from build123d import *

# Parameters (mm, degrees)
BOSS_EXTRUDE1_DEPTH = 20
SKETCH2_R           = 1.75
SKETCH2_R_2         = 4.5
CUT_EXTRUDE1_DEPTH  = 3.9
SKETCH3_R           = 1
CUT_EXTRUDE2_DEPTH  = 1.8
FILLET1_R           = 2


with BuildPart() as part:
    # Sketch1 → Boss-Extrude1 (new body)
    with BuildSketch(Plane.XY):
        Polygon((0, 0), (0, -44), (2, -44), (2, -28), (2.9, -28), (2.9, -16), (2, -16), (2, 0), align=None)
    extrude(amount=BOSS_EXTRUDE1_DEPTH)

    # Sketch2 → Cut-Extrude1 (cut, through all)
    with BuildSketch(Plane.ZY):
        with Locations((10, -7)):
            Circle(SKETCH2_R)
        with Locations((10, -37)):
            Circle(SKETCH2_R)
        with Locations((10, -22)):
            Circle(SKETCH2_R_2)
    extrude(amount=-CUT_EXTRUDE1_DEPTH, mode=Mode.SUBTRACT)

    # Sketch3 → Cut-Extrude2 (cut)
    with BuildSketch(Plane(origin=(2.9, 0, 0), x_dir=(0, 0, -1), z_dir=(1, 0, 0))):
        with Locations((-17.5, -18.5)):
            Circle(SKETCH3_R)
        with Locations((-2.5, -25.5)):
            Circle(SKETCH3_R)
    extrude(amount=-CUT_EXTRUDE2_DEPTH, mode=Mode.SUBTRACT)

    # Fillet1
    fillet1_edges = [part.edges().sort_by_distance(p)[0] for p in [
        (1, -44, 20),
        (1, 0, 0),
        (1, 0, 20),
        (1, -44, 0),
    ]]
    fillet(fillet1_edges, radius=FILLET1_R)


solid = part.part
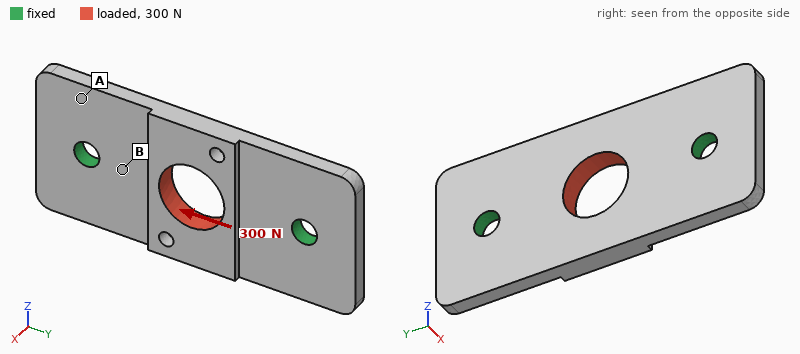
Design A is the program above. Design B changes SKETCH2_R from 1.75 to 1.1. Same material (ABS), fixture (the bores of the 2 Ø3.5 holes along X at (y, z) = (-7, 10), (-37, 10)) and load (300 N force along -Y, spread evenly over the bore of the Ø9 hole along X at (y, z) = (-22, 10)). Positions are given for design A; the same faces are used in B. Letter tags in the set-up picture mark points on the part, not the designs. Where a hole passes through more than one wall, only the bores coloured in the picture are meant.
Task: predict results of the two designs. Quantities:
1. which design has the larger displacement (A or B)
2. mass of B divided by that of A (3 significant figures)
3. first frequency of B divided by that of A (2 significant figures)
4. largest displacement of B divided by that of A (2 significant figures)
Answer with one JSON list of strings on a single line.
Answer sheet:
["B", "1.01", "0.86", "1.1"]
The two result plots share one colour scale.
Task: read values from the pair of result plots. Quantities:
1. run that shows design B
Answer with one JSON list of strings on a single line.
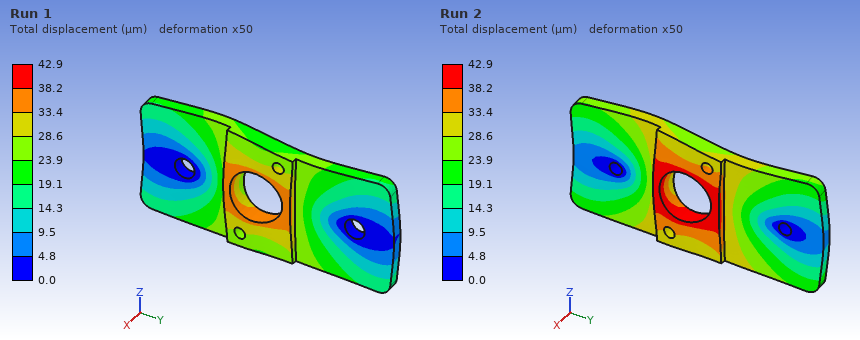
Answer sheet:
["Run 2"]
